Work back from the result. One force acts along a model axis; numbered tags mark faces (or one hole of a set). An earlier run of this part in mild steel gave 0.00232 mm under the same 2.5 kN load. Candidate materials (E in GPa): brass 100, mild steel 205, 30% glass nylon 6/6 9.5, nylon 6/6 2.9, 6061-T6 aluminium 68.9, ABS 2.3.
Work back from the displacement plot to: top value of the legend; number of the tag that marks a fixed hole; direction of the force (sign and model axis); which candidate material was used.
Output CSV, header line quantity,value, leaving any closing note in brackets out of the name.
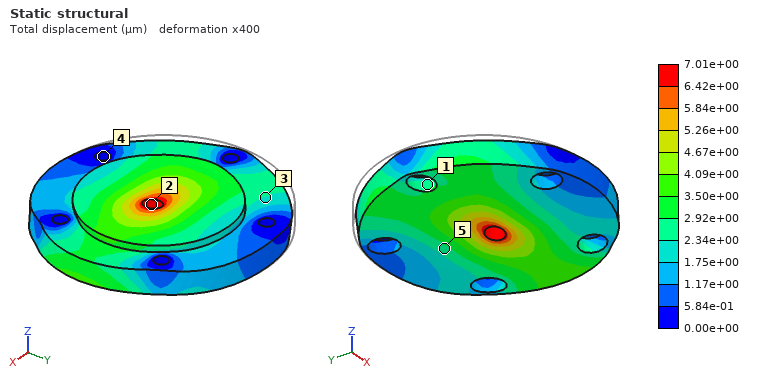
quantity,value
top value of the legend,7.01e+00 µm
number of the tag that marks a fixed hole,4
direction of the force,+X
which candidate material was used,6061-T6 aluminium
